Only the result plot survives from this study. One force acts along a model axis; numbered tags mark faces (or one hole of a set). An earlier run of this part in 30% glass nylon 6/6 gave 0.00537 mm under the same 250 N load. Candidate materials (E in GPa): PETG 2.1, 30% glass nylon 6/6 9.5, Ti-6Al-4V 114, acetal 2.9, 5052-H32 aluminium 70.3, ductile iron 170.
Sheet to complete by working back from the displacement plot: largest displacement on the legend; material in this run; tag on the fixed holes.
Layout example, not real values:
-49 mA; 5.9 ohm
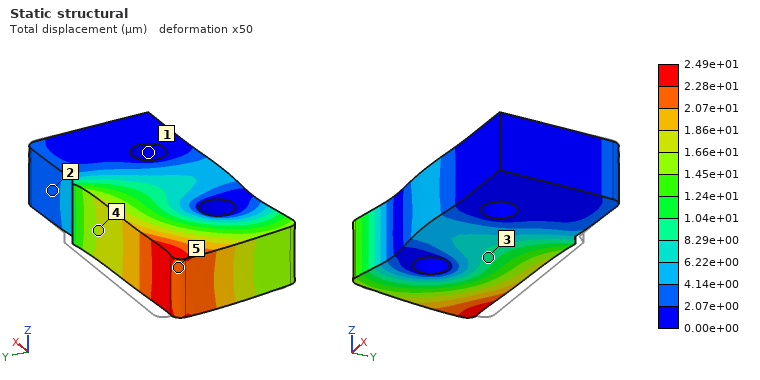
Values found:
2.49e+01 µm; PETG; 1
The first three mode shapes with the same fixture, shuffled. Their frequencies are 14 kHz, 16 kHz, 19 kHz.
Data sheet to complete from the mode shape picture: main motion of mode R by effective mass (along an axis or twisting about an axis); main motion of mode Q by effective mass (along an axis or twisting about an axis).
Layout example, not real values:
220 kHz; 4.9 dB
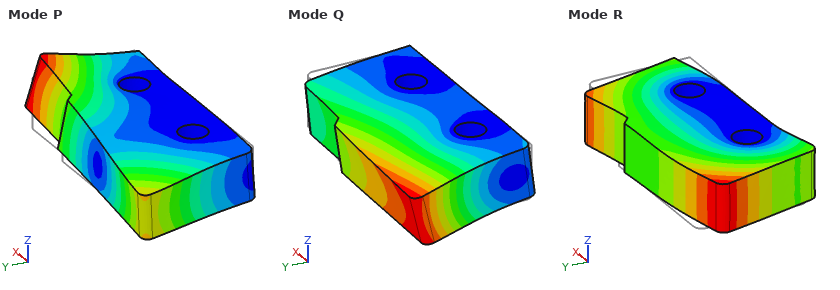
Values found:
along X; along Z
